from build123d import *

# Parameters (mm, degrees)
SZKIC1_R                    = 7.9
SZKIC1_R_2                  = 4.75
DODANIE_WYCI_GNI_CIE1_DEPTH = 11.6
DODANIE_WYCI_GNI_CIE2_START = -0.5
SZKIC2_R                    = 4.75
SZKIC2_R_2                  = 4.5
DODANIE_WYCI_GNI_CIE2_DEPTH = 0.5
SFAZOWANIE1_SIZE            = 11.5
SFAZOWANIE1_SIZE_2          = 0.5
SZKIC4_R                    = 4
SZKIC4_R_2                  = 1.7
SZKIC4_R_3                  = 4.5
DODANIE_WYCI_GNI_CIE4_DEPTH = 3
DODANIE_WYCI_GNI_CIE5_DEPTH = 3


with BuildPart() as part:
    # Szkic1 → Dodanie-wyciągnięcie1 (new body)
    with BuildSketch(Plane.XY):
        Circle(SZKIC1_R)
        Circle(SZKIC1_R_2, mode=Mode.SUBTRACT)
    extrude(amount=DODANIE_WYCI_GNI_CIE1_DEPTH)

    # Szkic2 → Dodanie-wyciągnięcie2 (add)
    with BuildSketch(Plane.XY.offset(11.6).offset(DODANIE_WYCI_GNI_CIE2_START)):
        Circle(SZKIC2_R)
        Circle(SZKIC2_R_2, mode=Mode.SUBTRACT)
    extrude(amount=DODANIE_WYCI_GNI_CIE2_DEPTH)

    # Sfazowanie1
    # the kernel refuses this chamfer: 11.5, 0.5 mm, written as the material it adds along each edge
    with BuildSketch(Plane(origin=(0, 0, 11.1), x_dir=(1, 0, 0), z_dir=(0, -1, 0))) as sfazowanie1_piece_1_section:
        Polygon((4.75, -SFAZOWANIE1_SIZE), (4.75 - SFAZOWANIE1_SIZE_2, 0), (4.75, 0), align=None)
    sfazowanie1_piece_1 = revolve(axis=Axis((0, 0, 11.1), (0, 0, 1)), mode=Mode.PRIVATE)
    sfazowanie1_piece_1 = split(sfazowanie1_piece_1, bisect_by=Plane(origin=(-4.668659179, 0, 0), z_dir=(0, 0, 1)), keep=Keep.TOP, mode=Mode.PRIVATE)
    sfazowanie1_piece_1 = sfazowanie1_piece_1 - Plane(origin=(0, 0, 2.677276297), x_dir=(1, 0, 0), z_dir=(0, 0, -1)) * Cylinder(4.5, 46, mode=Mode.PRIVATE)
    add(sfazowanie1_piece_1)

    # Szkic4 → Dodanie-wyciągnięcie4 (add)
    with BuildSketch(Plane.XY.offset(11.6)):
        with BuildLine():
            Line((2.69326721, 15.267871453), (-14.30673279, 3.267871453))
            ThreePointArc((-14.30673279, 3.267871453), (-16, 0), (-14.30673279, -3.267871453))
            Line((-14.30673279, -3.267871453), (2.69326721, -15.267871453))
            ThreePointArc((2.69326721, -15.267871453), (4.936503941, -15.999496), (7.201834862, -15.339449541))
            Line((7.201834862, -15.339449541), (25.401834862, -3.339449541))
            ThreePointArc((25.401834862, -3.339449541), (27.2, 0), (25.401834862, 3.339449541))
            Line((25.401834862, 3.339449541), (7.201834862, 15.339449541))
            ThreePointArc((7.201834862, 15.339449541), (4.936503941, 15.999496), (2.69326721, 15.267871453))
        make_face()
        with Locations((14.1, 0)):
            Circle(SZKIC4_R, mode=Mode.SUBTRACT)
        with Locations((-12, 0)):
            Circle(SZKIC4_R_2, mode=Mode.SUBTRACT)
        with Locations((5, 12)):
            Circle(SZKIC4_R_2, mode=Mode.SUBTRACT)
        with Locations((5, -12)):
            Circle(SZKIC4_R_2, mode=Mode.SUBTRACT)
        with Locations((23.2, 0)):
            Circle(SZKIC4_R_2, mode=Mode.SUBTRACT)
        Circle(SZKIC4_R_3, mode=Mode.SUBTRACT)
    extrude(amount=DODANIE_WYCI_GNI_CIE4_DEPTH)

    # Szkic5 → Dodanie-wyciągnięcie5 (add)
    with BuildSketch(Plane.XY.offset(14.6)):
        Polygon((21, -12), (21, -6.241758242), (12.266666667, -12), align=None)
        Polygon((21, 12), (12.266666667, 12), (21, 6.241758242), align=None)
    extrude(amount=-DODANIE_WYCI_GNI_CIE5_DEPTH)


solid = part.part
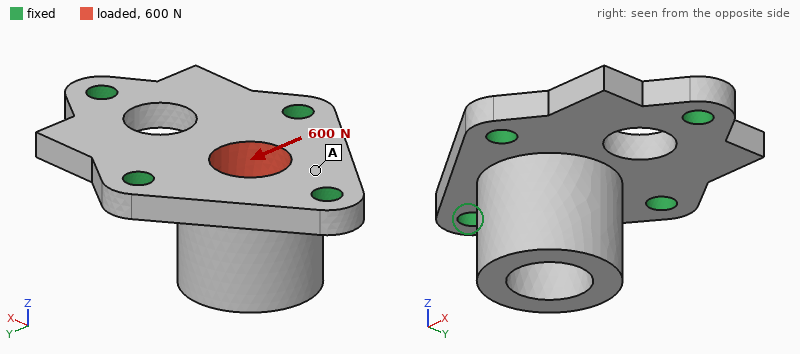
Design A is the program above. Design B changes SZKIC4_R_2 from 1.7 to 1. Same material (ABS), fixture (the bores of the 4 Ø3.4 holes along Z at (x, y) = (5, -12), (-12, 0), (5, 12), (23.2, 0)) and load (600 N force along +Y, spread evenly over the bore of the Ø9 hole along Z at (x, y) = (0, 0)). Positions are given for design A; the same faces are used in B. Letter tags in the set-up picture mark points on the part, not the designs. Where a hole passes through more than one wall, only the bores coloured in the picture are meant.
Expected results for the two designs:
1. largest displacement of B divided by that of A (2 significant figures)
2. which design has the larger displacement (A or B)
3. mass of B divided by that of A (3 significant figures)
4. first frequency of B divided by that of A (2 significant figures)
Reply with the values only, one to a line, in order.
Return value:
1.2
B
1.02
0.89
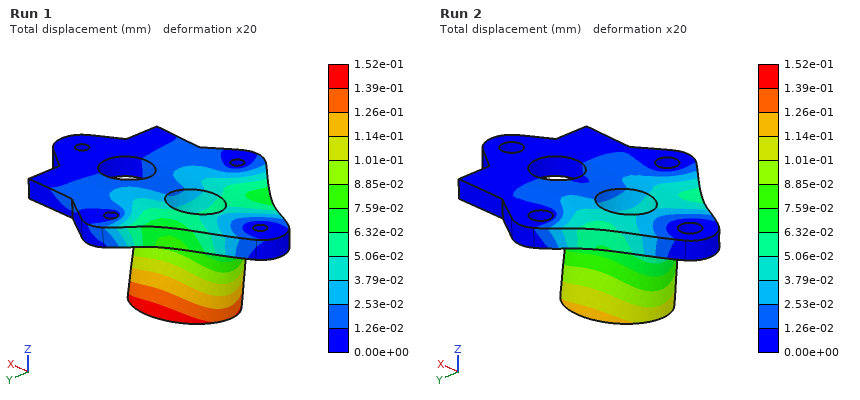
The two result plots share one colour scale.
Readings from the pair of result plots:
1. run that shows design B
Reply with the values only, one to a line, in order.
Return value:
Run 1
